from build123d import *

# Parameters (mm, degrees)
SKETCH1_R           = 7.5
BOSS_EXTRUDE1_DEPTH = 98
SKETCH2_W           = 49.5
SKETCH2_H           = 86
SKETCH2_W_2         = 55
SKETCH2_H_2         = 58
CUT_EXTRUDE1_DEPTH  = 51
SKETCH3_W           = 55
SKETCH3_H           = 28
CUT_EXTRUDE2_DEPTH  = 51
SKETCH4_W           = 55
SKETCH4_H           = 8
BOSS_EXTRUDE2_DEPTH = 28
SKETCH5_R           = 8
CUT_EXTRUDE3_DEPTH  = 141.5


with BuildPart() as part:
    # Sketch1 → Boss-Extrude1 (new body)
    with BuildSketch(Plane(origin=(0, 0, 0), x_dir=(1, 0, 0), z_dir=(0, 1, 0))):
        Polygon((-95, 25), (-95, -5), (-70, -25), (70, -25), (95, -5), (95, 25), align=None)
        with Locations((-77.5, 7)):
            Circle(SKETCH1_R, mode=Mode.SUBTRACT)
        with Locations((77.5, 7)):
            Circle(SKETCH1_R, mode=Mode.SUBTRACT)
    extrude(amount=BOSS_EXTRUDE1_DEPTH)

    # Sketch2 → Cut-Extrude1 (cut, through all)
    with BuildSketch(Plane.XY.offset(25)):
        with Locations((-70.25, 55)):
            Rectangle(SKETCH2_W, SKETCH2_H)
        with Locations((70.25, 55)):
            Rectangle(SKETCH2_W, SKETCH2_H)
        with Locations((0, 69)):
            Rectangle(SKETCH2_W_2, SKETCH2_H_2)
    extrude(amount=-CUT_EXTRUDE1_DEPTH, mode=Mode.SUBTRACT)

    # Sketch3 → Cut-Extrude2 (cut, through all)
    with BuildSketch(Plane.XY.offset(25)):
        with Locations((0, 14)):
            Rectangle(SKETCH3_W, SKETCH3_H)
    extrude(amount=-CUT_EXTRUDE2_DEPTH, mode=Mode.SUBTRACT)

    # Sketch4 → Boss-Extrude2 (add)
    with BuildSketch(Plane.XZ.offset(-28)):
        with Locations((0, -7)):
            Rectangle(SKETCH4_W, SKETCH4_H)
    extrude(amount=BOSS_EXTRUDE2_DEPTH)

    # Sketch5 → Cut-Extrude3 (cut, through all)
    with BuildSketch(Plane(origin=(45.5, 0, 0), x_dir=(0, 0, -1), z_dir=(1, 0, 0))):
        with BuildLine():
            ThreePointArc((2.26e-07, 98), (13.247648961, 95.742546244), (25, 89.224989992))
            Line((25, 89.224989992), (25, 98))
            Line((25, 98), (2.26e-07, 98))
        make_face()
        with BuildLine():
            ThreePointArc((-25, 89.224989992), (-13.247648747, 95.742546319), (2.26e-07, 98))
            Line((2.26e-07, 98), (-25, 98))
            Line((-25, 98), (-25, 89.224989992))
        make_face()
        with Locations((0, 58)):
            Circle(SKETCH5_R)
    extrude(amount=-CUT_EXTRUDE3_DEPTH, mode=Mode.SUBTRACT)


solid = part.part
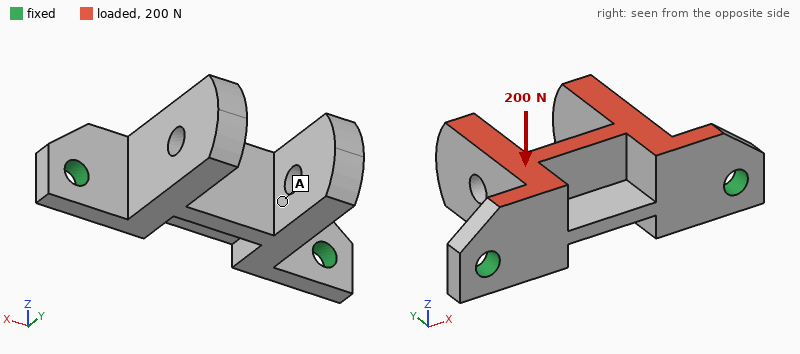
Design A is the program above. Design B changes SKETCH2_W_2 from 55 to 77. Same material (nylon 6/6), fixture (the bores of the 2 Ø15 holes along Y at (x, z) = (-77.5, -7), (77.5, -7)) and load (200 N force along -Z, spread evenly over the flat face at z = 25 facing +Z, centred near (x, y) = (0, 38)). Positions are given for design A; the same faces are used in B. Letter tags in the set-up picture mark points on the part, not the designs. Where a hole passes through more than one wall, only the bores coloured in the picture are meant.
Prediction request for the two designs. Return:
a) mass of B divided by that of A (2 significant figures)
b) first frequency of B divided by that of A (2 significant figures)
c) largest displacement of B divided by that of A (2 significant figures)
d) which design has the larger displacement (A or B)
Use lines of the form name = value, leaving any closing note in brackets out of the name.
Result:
mass of B divided by that of A = 0.78
first frequency of B divided by that of A = 1.4
largest displacement of B divided by that of A = 0.76
which design has the larger displacement = A
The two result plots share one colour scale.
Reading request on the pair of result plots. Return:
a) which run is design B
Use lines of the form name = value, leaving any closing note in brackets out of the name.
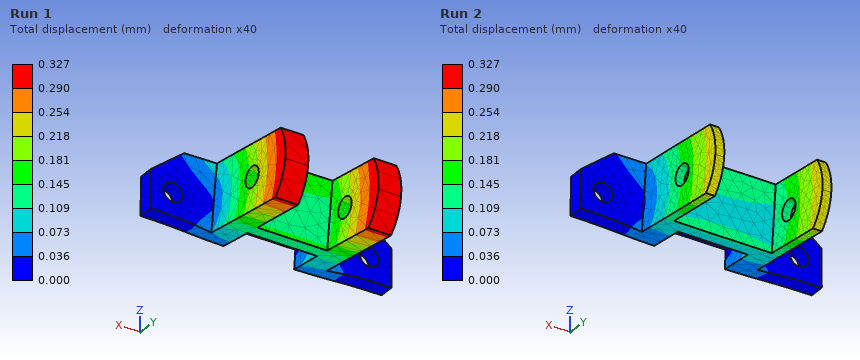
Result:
which run is design B = Run 2
